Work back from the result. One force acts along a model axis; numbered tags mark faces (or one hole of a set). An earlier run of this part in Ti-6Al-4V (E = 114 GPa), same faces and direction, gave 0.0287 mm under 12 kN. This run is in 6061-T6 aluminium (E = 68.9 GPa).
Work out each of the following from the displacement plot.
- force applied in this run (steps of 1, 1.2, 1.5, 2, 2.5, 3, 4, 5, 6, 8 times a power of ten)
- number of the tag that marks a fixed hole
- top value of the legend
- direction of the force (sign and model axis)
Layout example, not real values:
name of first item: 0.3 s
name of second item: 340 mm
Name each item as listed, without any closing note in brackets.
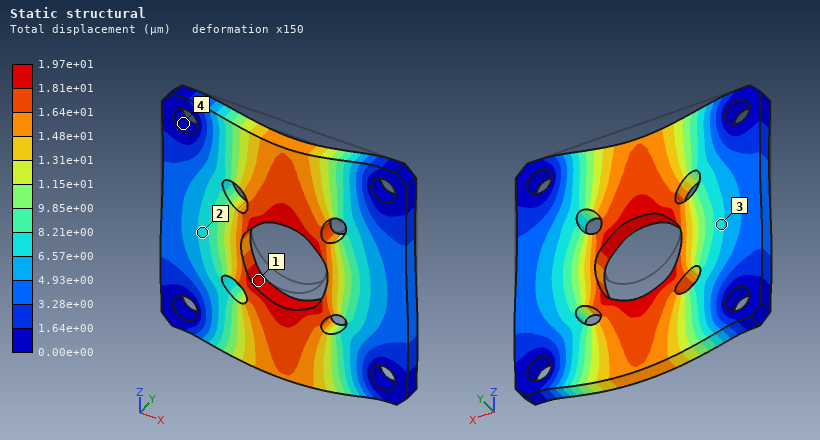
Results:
force applied in this run: 5 kN
number of the tag that marks a fixed hole: 4
top value of the legend: 1.97e+01 µm
direction of the force: -Z
